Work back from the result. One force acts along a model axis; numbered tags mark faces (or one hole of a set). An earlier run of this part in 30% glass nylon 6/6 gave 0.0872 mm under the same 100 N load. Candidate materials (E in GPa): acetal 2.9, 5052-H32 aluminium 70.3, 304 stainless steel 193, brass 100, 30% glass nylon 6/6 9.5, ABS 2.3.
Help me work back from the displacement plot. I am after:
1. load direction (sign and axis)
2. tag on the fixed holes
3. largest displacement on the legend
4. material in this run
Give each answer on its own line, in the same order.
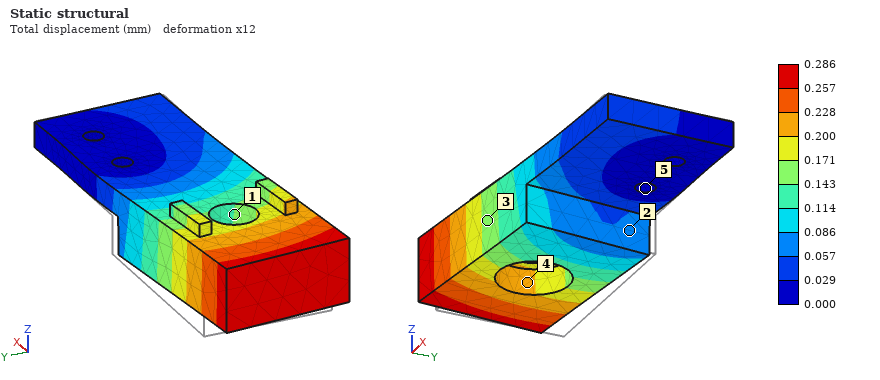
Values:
-Y
5
0.286 mm
acetal
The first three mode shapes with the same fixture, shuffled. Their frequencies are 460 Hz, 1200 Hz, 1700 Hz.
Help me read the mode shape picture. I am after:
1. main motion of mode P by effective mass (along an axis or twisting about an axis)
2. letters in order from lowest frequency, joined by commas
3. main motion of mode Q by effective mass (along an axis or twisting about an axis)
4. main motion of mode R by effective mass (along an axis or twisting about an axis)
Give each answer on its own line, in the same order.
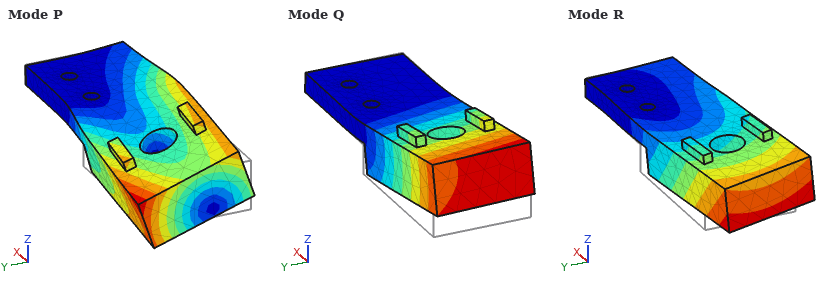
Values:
twisting about X
Q, R, P
along Z
along Y
